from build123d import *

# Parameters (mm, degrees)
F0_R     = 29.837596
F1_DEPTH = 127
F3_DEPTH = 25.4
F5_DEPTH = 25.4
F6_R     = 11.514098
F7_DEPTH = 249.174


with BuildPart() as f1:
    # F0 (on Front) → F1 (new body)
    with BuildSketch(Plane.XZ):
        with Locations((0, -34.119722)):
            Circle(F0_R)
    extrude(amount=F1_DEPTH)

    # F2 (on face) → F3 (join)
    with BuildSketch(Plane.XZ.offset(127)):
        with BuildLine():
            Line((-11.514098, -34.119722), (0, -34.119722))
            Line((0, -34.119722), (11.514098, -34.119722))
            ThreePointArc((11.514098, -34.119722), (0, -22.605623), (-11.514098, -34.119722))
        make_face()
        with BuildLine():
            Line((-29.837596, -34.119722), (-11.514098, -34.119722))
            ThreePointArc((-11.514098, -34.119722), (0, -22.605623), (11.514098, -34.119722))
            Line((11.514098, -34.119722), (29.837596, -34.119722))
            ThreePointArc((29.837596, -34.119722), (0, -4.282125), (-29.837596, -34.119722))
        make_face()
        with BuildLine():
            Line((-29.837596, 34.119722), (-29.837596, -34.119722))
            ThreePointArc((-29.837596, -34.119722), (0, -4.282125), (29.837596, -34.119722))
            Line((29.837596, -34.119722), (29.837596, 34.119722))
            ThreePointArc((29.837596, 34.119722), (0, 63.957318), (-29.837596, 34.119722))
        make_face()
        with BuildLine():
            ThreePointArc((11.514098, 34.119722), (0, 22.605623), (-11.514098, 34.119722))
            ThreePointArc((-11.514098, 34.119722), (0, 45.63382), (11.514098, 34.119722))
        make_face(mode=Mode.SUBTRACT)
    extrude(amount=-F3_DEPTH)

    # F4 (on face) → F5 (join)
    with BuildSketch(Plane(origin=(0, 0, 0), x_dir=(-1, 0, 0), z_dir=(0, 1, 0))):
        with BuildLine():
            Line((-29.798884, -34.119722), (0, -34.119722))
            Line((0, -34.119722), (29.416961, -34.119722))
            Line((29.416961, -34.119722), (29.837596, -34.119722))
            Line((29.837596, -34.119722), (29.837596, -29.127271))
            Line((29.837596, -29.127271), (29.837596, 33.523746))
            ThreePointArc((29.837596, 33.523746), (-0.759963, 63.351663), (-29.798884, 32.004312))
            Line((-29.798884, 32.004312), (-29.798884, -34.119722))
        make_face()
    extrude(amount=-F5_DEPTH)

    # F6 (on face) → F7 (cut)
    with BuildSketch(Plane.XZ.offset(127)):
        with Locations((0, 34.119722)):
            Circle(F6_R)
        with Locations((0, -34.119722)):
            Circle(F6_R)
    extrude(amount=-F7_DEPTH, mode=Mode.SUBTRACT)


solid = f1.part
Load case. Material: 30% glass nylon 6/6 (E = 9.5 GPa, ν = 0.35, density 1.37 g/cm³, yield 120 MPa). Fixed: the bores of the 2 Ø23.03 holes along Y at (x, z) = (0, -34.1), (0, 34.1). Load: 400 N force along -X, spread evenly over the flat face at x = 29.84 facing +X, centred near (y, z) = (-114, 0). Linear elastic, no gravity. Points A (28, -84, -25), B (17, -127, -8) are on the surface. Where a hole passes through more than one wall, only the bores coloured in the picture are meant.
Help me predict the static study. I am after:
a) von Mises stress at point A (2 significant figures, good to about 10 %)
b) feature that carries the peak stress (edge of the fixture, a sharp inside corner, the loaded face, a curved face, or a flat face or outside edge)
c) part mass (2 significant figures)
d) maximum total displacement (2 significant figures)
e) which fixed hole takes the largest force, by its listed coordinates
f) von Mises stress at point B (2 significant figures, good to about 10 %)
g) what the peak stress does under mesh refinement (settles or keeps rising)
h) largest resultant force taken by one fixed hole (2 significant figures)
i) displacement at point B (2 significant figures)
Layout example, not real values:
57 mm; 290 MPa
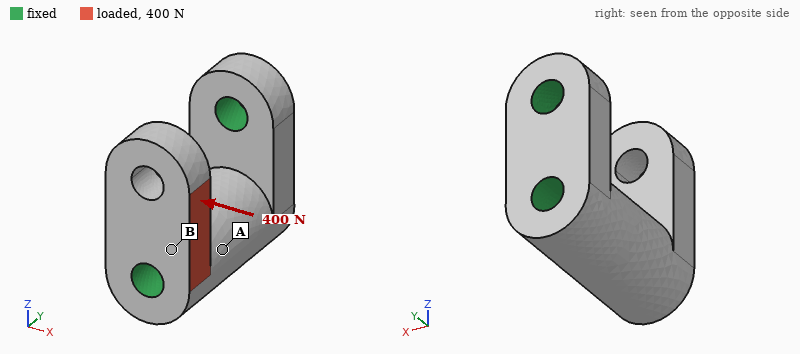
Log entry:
0.17 MPa; edge of the fixture; 670 g; 10 µm; (0, -34.1); 0.39 MPa; keeps rising; 400 N; 2.9 µm
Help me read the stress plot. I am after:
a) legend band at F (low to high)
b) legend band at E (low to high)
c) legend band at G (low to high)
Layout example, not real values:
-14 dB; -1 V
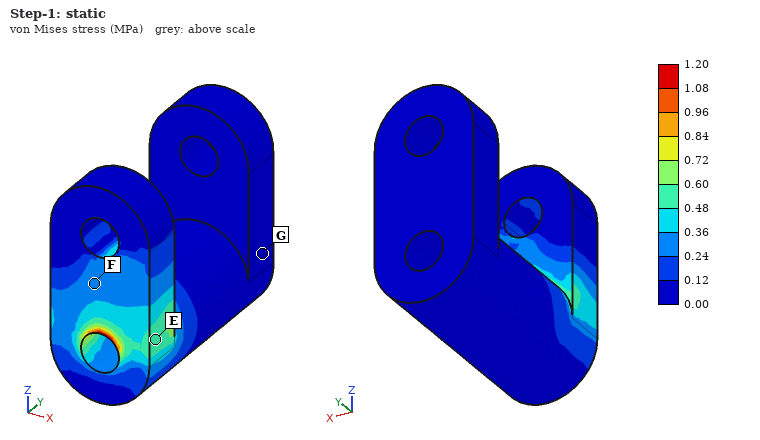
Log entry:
0.24 to 0.36 MPa; 0.48 to 0.60 MPa; 0.00 to 0.12 MPa
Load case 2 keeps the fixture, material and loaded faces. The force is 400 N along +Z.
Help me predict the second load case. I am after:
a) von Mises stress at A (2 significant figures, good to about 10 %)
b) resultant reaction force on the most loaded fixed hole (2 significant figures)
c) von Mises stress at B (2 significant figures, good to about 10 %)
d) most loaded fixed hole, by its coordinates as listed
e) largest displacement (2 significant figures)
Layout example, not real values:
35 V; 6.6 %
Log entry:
0.14 MPa; 400 N; 0.49 MPa; (0, -34.1); 9.9 µm
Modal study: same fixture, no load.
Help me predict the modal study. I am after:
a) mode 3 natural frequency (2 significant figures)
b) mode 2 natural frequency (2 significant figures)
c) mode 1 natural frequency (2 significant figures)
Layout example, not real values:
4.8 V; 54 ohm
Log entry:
3900 Hz; 2300 Hz; 1800 Hz
